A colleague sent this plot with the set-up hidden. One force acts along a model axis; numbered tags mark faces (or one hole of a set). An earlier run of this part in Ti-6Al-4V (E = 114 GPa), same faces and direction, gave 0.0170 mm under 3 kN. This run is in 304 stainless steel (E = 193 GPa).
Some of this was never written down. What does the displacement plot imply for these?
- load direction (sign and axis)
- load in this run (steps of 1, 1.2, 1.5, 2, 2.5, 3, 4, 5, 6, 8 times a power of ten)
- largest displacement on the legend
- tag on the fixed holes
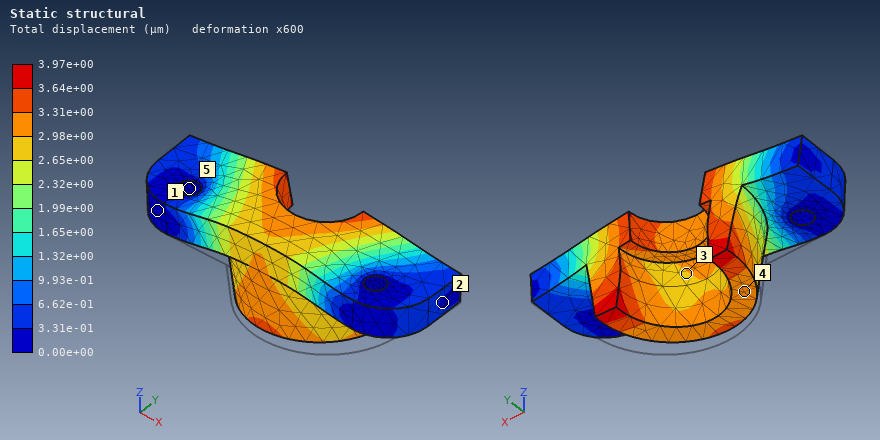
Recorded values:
+Z
1.2 kN
3.97e+00 µm
5
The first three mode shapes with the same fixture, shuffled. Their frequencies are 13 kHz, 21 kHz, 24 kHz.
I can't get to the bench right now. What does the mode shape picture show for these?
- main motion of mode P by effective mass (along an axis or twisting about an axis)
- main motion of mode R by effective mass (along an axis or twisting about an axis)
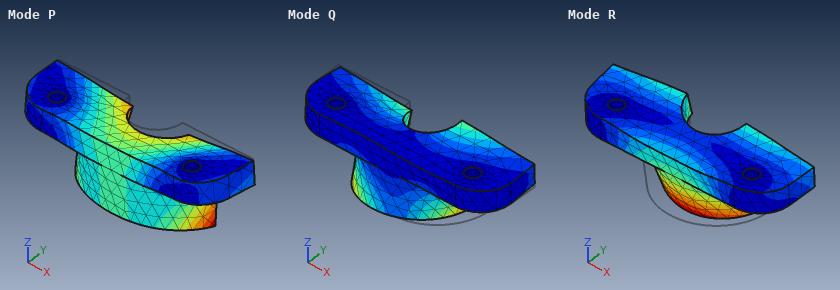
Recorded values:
along Z
along Y
